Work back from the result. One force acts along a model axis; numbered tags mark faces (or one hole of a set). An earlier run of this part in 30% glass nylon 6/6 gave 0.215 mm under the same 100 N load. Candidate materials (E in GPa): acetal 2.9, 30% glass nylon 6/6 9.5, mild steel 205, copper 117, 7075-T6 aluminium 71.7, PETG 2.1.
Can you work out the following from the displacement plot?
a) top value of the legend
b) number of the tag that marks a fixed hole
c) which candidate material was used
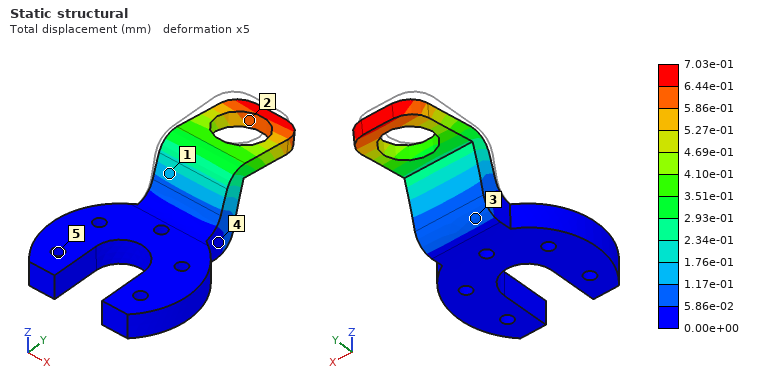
7.03e-01 mm
5
acetal
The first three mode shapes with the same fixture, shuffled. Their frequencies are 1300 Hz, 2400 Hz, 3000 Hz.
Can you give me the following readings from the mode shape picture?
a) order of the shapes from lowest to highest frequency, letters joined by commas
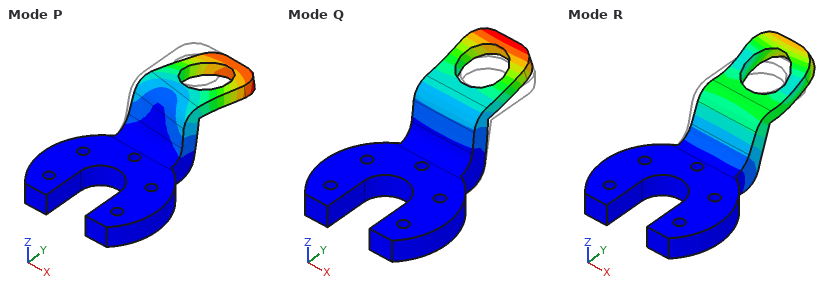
Q, P, R
